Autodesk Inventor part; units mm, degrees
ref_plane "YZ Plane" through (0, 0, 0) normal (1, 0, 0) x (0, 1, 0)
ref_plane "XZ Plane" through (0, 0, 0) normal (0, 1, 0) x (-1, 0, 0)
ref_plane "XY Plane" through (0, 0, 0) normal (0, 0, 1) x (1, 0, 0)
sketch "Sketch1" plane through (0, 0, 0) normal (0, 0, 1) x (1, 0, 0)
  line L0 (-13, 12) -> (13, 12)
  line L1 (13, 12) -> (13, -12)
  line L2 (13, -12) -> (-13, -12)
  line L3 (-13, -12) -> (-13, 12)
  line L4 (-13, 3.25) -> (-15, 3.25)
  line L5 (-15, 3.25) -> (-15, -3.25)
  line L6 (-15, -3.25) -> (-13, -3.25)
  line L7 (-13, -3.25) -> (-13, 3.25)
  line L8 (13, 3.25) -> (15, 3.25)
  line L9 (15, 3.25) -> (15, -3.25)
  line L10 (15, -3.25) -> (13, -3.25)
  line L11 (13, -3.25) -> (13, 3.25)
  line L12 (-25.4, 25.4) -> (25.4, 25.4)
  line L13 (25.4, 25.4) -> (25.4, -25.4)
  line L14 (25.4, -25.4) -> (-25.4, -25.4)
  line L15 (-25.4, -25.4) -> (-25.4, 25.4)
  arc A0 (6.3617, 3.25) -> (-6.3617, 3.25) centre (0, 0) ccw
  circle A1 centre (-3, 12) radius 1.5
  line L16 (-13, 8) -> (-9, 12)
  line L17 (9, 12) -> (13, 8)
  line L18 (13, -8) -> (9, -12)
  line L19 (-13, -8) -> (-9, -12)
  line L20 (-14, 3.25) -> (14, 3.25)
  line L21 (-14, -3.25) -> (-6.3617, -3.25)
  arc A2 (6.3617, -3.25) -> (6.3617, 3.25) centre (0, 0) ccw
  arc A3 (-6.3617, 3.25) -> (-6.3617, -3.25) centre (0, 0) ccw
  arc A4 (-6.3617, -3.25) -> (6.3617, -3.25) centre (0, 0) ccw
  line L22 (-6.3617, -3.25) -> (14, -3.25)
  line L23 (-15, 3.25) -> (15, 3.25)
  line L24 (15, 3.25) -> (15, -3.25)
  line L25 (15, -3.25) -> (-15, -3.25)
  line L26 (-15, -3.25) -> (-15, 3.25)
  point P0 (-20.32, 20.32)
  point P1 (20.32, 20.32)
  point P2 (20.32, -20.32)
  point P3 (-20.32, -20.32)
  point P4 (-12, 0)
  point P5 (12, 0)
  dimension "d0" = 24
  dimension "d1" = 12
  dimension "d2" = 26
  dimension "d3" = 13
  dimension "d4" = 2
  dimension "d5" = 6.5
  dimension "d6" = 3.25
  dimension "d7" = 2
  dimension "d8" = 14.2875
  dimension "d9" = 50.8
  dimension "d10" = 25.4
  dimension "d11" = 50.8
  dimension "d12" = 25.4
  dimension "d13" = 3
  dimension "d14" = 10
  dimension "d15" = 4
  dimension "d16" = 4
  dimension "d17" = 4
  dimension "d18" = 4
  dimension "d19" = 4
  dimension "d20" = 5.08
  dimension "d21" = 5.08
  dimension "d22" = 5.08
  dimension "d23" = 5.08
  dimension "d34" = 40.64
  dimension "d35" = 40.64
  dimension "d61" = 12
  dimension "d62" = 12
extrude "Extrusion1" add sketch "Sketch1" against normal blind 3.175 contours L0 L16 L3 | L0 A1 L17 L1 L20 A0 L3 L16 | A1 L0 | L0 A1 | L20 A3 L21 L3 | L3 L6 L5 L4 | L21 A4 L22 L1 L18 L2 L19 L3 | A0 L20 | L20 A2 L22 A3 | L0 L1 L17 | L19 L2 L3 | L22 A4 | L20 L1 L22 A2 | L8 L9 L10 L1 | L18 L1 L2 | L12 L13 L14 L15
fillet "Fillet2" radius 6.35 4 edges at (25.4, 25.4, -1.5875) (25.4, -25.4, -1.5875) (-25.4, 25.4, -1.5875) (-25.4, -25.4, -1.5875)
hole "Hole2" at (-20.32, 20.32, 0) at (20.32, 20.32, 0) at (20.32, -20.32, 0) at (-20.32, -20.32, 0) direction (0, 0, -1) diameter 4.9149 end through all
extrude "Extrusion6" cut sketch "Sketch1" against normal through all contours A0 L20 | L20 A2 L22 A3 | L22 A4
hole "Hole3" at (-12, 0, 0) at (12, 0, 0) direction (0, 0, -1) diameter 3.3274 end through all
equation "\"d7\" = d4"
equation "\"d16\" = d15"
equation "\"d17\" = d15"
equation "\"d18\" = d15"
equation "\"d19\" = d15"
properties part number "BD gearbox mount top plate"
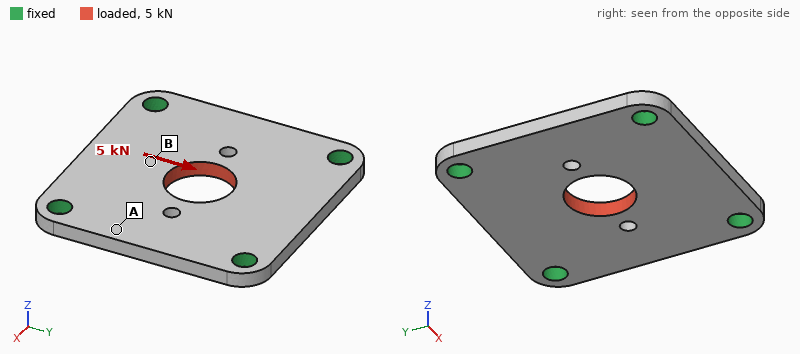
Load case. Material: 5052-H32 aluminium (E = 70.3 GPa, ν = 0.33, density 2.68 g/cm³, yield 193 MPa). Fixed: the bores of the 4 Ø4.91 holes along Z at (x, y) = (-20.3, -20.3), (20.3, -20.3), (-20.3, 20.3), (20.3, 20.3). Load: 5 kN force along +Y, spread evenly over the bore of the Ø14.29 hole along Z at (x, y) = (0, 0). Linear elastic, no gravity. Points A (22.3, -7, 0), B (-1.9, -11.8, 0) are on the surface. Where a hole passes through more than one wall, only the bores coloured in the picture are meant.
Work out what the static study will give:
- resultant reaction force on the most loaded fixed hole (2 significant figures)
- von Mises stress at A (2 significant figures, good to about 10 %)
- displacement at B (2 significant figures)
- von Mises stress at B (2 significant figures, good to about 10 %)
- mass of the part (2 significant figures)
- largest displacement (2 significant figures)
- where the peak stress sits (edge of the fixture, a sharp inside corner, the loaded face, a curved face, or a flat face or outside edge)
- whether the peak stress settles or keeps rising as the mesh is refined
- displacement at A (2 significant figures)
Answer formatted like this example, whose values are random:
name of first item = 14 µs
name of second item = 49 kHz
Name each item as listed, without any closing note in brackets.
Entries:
resultant reaction force on the most loaded fixed hole = 1.4 kN
von Mises stress at A = 11 MPa
displacement at B = 13 µm
von Mises stress at B = 25 MPa
mass of the part = 20 g
largest displacement = 15 µm
where the peak stress sits = edge of the fixture
whether the peak stress settles or keeps rising as the mesh is refined = keeps rising
displacement at A = 3.0 µm
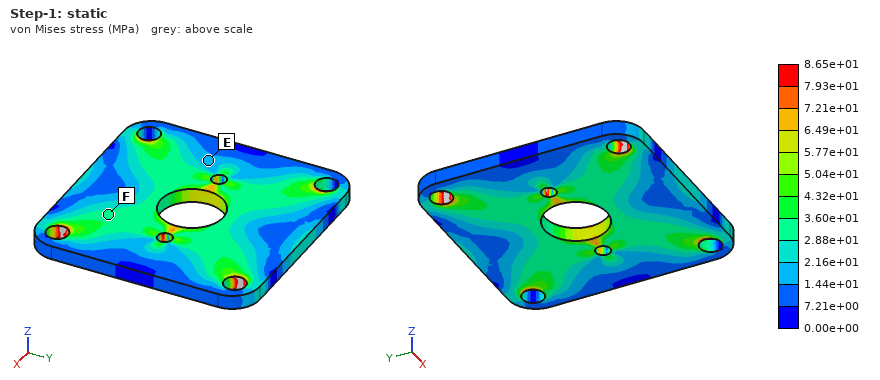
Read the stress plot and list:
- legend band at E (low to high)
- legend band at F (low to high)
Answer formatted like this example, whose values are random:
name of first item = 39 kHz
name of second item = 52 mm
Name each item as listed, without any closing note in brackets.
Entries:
legend band at E = 1.44e+01 to 2.16e+01 MPa
legend band at F = 2.88e+01 to 3.60e+01 MPa
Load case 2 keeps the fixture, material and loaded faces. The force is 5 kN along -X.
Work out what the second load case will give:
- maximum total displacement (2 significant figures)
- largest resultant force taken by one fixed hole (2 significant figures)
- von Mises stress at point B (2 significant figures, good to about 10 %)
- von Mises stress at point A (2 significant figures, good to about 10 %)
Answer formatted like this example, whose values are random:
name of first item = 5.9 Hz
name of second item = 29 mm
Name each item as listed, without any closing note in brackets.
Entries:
maximum total displacement = 16 µm
largest resultant force taken by one fixed hole = 1.4 kN
von Mises stress at point B = 34 MPa
von Mises stress at point A = 12 MPa
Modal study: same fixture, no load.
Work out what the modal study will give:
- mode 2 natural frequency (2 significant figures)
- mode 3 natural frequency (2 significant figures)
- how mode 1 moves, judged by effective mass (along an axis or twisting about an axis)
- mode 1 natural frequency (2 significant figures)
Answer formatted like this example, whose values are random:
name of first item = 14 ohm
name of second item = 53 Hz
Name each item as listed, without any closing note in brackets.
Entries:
mode 2 natural frequency = 12 kHz
mode 3 natural frequency = 12 kHz
how mode 1 moves, judged by effective mass = along Z
mode 1 natural frequency = 7800 Hz
